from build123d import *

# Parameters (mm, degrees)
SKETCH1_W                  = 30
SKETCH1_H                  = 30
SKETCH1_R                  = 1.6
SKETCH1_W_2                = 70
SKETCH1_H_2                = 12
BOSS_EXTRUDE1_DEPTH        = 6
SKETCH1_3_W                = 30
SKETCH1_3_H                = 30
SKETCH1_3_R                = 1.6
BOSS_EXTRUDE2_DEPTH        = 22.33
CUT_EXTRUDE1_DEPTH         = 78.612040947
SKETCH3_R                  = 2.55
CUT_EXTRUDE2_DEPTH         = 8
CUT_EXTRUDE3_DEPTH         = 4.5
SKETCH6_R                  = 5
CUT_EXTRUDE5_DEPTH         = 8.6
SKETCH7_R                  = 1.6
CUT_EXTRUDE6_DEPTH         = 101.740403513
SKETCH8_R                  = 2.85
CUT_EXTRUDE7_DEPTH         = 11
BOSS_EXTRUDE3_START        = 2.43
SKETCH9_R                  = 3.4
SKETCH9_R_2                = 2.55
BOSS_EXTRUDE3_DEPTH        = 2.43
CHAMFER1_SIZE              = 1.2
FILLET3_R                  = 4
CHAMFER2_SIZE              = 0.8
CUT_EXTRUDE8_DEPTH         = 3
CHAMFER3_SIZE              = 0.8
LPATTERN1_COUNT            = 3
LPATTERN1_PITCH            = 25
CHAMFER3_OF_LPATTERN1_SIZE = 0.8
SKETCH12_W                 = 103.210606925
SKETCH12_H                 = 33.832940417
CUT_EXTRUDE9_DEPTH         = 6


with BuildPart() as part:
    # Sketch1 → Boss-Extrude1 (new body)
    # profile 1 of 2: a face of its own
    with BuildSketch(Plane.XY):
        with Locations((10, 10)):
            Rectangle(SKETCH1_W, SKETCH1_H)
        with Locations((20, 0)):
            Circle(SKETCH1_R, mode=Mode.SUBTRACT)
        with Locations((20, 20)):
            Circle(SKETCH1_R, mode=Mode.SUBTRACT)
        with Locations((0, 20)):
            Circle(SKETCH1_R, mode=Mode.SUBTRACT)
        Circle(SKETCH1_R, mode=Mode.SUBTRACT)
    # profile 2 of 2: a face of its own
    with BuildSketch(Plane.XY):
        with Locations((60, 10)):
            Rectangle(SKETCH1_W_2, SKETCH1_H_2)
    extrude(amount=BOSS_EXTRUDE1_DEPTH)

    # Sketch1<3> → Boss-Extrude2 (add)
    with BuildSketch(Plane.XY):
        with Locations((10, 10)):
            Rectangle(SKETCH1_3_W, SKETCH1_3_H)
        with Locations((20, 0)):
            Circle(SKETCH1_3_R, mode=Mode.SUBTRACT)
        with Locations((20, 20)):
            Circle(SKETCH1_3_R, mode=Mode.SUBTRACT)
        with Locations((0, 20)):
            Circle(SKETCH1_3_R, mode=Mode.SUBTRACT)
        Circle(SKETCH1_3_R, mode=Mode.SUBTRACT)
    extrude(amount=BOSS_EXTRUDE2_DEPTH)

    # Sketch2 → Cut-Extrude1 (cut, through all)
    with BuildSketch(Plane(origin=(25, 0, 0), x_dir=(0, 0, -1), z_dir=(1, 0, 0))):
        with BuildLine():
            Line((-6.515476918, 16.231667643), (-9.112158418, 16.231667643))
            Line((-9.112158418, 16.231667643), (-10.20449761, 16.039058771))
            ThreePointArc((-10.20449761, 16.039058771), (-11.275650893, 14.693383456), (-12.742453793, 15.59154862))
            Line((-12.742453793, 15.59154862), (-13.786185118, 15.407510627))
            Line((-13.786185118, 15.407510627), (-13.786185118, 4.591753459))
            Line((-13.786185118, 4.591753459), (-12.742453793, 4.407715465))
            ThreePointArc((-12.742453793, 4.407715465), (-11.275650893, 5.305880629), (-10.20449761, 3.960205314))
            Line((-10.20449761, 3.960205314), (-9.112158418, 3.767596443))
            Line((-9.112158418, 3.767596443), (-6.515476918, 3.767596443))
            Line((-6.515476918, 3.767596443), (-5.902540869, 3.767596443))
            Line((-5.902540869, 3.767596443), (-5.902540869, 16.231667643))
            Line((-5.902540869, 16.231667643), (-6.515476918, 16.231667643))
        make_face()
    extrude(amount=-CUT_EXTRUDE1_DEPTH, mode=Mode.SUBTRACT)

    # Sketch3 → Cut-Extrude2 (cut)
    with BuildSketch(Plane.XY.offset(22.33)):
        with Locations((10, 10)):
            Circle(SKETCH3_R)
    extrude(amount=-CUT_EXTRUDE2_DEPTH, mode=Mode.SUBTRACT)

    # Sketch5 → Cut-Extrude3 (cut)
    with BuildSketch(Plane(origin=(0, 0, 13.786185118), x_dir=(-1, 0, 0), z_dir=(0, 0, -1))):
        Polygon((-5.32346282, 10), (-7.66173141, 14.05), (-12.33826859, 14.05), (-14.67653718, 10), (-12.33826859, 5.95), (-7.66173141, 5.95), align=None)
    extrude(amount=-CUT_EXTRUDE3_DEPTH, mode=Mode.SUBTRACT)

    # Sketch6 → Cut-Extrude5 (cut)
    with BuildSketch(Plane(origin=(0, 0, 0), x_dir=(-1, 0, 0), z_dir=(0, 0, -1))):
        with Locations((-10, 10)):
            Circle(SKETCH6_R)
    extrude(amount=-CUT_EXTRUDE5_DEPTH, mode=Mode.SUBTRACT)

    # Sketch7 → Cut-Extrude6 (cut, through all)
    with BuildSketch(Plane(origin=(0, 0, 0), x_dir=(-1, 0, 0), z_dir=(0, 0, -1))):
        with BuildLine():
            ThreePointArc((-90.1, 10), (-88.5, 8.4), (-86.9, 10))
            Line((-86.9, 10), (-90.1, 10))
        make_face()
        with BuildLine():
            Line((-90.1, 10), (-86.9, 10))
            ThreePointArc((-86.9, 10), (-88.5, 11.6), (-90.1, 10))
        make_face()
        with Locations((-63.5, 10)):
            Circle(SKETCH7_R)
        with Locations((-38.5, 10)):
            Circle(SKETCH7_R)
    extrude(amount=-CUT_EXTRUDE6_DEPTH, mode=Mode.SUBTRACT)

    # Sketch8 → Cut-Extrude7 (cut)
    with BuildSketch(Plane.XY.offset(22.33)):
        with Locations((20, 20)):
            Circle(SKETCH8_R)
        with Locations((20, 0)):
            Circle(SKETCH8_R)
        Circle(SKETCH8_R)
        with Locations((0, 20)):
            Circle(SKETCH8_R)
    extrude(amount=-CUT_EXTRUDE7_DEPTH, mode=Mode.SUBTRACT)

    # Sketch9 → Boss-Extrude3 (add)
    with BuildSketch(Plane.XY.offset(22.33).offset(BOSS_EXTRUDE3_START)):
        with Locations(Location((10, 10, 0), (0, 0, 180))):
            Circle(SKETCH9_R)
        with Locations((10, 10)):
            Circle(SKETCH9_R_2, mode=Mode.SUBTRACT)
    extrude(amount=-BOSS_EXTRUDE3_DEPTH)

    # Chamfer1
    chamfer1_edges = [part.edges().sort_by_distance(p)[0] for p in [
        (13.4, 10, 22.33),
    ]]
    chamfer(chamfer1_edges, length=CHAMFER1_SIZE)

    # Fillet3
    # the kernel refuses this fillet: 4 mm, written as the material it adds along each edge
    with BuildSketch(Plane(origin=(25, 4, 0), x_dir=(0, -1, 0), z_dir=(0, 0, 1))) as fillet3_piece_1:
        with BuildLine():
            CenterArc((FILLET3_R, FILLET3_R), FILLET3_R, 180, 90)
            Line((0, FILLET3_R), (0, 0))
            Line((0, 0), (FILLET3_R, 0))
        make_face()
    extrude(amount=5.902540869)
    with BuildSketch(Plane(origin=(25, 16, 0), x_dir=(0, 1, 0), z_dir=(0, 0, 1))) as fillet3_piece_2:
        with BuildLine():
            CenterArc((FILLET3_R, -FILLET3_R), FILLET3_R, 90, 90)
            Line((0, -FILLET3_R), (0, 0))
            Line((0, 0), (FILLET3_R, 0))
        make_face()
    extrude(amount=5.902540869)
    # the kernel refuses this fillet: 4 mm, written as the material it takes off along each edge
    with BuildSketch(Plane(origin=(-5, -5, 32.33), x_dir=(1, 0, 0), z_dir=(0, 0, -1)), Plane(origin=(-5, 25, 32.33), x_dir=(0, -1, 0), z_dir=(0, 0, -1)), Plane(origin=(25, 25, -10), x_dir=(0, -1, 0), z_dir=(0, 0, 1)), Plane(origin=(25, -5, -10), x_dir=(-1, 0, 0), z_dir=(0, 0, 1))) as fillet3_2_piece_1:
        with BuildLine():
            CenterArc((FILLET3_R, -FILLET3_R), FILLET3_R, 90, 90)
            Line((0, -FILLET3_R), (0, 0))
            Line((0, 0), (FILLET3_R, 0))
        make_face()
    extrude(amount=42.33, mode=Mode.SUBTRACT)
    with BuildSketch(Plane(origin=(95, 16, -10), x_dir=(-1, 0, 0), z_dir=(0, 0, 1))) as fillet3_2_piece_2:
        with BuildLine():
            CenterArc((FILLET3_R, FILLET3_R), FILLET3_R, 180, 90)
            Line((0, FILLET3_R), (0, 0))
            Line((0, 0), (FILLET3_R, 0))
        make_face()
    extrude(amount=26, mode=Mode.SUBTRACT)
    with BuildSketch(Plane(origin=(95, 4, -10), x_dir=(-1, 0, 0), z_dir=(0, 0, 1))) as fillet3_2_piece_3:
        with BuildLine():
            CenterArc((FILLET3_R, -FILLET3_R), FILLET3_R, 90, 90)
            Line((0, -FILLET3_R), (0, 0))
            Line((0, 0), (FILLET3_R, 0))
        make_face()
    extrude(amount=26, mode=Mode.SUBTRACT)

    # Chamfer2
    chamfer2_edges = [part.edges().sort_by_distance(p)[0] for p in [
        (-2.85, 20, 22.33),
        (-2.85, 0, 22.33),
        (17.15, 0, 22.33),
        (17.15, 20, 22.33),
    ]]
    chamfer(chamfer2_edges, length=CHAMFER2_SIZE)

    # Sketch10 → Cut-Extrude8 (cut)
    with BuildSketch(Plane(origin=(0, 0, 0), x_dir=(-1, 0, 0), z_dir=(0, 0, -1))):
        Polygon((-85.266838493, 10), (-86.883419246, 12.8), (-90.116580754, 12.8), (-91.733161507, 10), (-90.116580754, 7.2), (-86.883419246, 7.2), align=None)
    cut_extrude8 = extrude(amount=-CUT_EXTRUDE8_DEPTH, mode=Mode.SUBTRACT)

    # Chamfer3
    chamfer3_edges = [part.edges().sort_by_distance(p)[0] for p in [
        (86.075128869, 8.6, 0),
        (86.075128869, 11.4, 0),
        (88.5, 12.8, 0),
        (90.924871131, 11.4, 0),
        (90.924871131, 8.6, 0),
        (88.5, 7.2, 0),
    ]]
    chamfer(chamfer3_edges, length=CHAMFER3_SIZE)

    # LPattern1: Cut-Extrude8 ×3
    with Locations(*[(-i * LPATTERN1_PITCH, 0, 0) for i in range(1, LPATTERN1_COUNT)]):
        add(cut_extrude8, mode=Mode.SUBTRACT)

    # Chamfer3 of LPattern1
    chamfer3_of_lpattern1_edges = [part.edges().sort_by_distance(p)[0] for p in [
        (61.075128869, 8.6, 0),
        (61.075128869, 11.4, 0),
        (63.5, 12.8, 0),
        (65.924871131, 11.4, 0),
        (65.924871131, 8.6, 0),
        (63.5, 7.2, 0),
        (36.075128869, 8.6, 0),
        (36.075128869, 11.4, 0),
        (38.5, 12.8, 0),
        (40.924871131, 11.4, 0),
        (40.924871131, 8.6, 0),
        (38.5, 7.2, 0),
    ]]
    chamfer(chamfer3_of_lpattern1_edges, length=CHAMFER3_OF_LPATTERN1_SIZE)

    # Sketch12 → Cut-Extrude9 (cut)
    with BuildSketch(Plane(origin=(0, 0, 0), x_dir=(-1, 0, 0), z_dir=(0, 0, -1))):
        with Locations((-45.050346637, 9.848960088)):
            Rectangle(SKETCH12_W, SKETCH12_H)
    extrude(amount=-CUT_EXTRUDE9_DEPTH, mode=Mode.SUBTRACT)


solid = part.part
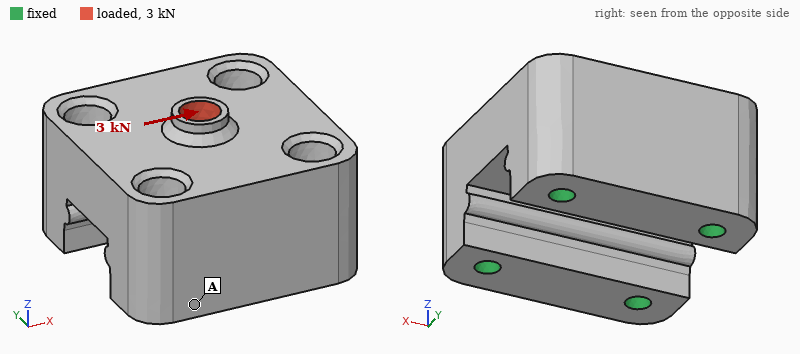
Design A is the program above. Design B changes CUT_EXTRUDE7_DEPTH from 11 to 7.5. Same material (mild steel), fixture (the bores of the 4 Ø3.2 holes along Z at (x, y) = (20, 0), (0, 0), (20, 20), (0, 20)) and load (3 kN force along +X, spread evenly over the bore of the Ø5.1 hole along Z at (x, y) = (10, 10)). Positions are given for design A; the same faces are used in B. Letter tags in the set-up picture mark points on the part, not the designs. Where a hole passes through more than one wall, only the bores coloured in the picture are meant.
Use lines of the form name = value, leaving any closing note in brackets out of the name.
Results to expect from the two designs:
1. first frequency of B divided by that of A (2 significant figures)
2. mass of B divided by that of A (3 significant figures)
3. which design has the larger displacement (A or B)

first frequency of B divided by that of A = 1.6
mass of B divided by that of A = 1.02
which design has the larger displacement = A
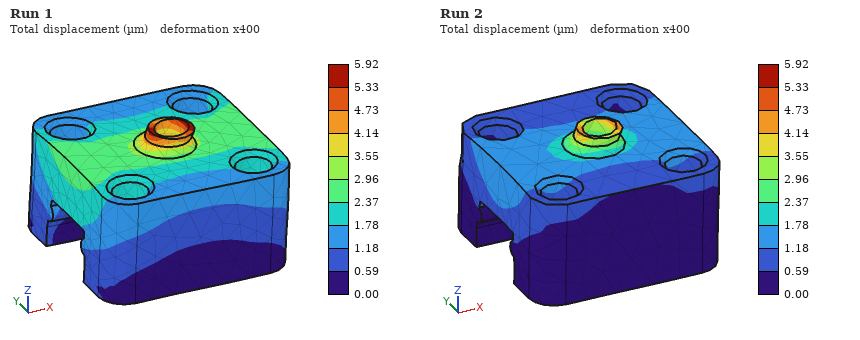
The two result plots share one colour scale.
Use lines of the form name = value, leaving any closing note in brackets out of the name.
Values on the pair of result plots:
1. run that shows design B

run that shows design B = Run 2
